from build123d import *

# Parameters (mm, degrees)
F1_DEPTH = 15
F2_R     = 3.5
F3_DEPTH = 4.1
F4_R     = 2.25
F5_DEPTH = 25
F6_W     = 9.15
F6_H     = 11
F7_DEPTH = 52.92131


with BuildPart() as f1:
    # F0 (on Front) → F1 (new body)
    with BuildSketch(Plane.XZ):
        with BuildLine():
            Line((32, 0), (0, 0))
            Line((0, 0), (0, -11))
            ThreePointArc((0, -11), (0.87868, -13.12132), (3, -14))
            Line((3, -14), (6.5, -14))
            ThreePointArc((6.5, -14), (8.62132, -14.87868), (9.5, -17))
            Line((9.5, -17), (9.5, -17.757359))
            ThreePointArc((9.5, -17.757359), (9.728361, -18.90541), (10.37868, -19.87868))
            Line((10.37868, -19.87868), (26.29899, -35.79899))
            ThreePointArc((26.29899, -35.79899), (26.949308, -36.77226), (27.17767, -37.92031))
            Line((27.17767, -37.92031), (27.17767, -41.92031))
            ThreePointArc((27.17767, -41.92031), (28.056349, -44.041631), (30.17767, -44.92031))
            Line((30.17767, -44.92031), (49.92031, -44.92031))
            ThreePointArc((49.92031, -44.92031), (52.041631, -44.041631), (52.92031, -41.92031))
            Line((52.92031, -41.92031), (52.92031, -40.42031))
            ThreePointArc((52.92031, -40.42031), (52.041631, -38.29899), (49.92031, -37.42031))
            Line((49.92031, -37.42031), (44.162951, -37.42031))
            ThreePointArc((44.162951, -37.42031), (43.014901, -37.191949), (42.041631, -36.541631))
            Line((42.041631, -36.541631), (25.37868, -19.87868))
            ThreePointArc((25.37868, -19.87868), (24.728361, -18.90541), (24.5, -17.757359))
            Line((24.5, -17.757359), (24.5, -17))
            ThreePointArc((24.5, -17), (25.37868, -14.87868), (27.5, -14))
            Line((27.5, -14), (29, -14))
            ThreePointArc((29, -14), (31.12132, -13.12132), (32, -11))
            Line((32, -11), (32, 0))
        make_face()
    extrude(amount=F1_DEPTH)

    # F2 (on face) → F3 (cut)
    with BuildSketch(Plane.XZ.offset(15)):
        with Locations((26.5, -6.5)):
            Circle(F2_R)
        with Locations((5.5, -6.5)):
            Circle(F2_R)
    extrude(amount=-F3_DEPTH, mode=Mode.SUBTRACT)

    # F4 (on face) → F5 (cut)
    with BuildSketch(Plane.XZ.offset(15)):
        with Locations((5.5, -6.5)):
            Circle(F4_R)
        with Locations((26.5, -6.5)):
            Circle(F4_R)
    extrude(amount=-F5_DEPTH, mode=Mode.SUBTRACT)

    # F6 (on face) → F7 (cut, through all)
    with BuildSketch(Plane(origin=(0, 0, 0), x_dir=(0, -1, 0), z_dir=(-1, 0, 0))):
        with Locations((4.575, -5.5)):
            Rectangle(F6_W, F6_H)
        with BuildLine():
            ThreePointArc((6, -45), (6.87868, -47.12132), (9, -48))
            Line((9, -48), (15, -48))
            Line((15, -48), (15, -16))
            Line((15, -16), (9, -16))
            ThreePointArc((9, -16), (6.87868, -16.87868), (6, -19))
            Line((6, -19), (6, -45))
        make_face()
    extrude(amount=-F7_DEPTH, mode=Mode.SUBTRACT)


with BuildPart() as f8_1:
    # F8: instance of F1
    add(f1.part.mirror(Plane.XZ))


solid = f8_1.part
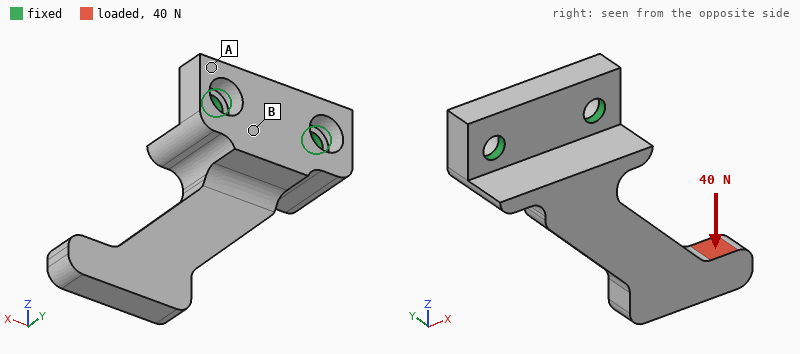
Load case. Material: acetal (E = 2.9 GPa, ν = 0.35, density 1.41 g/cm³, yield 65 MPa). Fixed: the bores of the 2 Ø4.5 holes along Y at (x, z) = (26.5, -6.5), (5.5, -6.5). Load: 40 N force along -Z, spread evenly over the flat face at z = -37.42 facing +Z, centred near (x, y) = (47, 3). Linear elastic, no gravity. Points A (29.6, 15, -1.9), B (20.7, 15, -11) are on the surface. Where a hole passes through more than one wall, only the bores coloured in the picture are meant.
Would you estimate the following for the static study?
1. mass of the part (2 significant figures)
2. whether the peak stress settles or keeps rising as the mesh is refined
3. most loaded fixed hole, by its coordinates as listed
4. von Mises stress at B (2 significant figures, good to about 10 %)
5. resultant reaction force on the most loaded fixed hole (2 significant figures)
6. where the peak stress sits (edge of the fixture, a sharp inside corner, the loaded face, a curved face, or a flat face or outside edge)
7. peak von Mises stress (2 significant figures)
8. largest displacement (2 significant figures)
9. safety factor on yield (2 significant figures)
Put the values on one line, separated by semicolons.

9.4 g; settles; (26.5, -6.5); 3.0 MPa; 80 N; a curved face; 23 MPa; 0.77 mm; 2.8
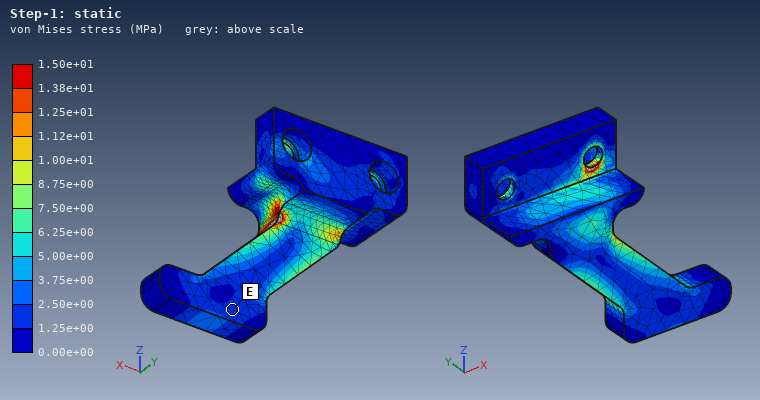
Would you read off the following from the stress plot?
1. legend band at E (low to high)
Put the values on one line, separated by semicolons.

1.25e+00 to 2.50e+00 MPa
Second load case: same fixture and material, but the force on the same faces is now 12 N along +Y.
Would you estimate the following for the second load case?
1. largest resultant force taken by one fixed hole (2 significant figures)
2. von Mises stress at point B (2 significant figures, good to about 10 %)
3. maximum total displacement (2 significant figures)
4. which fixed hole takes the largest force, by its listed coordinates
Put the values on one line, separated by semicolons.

23 N; 2.7 MPa; 0.78 mm; (26.5, -6.5)
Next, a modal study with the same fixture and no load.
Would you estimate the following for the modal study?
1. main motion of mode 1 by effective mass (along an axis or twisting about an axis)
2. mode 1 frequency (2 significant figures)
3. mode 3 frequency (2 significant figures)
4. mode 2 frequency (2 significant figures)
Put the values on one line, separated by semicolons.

along Y; 480 Hz; 1800 Hz; 1000 Hz
